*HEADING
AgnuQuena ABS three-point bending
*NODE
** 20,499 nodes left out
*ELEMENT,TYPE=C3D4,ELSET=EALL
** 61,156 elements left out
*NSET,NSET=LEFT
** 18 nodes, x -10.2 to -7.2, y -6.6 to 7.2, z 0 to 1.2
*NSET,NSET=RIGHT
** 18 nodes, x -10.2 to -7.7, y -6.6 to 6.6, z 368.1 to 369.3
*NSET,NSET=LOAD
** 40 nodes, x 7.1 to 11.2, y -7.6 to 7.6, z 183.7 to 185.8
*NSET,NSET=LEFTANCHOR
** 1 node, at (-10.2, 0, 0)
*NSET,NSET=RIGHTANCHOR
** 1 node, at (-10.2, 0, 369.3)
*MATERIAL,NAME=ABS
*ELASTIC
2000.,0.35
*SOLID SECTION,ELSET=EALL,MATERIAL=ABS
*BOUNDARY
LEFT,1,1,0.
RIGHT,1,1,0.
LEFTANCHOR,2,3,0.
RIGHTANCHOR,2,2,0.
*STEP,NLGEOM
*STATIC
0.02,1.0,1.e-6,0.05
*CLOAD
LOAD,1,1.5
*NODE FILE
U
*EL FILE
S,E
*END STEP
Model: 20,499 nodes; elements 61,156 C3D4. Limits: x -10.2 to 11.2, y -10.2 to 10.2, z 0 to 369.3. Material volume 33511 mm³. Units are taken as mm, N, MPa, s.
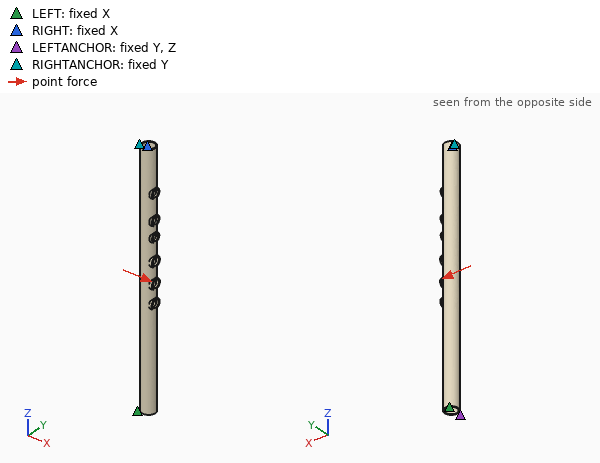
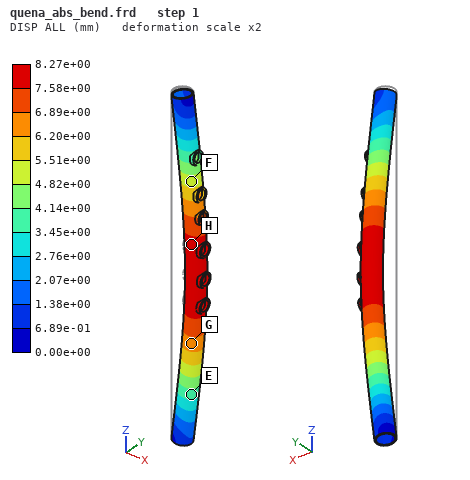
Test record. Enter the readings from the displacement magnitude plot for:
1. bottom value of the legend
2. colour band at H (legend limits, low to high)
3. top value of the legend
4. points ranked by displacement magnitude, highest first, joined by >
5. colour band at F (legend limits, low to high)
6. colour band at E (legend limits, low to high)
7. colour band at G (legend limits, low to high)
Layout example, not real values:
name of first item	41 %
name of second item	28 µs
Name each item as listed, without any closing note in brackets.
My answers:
bottom value of the legend	0.00e+00 mm
colour band at H	7.58e+00 to 8.27e+00 mm
top value of the legend	8.27e+00 mm
points ranked by displacement magnitude, highest first, joined by >	H > G > F > E
colour band at F	4.82e+00 to 5.51e+00 mm
colour band at E	3.45e+00 to 4.14e+00 mm
colour band at G	6.20e+00 to 6.89e+00 mm
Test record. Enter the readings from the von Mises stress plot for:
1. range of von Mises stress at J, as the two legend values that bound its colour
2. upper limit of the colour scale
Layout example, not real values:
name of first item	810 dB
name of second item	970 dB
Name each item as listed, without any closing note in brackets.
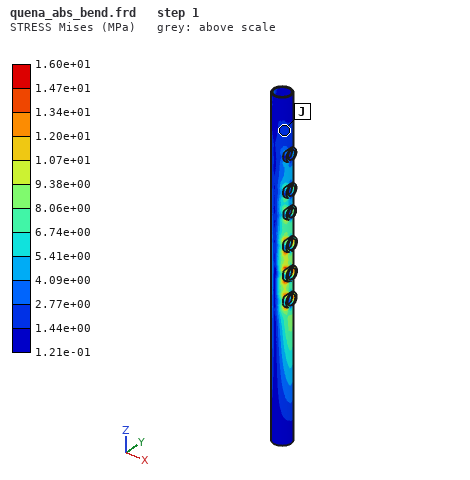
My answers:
range of von Mises stress at J, as the two legend values that bound its colour	1.44e+00 to 2.77e+00 MPa
upper limit of the colour scale	1.60e+01 MPa
